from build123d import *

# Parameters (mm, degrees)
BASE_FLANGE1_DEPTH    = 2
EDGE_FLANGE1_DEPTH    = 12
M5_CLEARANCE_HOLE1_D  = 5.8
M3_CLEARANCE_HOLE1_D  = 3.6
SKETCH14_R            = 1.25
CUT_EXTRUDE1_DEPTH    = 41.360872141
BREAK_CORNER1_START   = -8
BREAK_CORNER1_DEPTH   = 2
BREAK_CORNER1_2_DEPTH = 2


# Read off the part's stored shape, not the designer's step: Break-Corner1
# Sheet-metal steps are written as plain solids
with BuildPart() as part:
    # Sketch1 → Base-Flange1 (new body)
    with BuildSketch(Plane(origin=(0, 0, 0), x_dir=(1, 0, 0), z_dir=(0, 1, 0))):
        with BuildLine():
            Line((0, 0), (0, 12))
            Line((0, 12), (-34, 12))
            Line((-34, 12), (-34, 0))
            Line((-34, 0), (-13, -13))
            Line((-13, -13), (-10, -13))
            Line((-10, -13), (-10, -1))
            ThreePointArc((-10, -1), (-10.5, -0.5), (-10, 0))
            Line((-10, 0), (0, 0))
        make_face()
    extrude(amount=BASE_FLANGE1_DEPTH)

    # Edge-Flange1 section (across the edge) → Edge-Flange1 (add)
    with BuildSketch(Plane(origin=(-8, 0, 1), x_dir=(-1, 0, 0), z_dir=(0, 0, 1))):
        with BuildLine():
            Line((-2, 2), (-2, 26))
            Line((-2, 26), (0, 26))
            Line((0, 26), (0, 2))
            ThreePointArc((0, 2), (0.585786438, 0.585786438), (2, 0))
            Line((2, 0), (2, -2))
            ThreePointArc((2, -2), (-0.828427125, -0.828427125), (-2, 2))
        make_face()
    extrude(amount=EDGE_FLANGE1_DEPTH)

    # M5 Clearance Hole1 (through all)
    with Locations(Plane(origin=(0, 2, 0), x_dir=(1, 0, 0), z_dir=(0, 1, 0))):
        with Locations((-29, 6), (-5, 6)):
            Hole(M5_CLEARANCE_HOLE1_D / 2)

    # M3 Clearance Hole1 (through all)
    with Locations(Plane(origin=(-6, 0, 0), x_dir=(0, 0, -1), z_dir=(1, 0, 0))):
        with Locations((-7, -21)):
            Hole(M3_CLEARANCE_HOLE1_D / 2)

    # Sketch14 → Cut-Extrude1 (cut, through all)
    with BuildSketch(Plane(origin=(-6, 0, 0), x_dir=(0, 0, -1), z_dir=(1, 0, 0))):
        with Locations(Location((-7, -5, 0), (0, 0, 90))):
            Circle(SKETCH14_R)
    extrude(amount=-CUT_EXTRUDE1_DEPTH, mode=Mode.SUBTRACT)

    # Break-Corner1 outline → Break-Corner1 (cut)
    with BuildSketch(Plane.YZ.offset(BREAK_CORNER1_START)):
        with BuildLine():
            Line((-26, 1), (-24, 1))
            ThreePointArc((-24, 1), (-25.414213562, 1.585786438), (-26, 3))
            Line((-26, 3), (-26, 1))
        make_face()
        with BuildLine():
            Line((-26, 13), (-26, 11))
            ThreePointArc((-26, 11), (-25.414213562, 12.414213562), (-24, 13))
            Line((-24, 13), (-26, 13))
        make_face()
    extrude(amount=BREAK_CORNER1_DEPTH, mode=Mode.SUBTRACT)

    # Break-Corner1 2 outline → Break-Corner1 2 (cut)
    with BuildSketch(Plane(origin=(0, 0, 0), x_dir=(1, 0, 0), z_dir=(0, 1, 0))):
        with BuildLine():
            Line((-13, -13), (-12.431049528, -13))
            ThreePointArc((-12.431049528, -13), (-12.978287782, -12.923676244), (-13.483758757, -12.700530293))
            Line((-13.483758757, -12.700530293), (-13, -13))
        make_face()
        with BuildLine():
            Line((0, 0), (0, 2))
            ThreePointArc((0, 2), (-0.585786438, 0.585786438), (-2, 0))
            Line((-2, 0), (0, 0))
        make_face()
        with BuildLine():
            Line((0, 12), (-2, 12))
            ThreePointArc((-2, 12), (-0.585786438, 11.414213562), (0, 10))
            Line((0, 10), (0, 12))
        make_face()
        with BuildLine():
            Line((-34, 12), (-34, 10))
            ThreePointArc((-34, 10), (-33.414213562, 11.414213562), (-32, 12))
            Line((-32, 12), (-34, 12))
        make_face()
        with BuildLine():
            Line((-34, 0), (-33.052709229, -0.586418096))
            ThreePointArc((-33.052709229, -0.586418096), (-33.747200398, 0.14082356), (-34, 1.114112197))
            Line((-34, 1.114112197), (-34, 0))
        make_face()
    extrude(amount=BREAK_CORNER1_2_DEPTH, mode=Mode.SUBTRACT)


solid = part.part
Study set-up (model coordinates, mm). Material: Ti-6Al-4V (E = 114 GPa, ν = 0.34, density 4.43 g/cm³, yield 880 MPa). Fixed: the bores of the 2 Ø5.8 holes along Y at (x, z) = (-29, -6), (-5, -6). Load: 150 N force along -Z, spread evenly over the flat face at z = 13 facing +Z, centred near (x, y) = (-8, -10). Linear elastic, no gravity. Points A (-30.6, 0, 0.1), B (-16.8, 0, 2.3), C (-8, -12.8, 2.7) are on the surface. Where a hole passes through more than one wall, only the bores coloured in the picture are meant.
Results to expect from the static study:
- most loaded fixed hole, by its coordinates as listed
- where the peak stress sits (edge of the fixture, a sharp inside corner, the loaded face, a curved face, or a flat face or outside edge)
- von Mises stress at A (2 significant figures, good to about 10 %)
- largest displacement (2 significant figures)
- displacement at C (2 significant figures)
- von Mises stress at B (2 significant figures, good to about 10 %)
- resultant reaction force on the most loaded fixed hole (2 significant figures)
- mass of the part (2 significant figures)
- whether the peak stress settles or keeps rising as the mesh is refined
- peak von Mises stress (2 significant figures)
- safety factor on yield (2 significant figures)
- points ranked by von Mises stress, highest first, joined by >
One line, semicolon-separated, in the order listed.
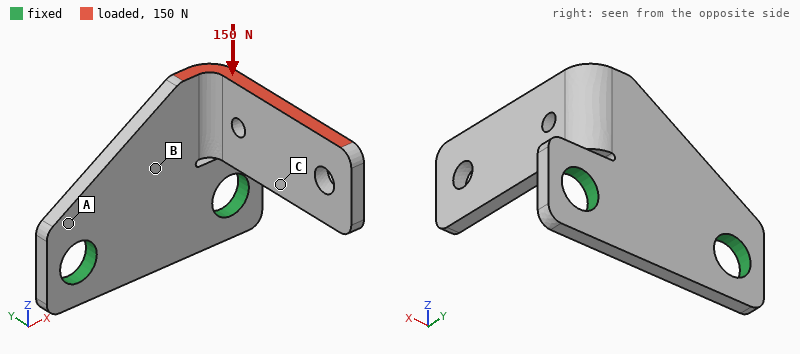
(-5, -6); a curved face; 62 MPa; 0.60 mm; 0.29 mm; 140 MPa; 140 N; 7.6 g; settles; 810 MPa; 1.1; B > A > C
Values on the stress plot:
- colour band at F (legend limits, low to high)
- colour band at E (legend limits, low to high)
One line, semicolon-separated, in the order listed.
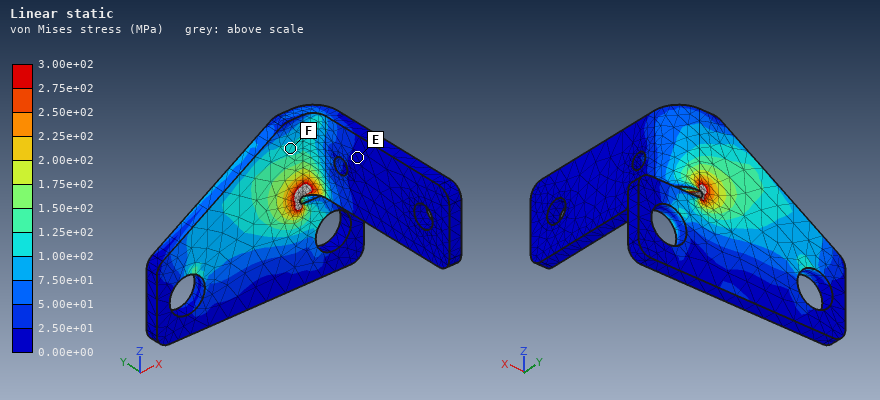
1.00e+02 to 1.25e+02 MPa; 0.00e+00 to 2.50e+01 MPa
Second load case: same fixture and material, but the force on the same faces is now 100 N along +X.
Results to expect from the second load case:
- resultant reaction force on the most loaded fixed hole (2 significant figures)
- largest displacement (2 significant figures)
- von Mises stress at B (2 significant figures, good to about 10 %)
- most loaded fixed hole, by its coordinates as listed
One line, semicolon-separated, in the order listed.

120 N; 0.52 mm; 65 MPa; (-29, -6)
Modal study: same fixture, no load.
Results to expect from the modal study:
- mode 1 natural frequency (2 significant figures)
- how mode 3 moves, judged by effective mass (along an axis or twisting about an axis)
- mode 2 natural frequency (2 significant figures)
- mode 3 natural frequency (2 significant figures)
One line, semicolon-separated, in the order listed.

1400 Hz; along Y; 1700 Hz; 5700 Hz
